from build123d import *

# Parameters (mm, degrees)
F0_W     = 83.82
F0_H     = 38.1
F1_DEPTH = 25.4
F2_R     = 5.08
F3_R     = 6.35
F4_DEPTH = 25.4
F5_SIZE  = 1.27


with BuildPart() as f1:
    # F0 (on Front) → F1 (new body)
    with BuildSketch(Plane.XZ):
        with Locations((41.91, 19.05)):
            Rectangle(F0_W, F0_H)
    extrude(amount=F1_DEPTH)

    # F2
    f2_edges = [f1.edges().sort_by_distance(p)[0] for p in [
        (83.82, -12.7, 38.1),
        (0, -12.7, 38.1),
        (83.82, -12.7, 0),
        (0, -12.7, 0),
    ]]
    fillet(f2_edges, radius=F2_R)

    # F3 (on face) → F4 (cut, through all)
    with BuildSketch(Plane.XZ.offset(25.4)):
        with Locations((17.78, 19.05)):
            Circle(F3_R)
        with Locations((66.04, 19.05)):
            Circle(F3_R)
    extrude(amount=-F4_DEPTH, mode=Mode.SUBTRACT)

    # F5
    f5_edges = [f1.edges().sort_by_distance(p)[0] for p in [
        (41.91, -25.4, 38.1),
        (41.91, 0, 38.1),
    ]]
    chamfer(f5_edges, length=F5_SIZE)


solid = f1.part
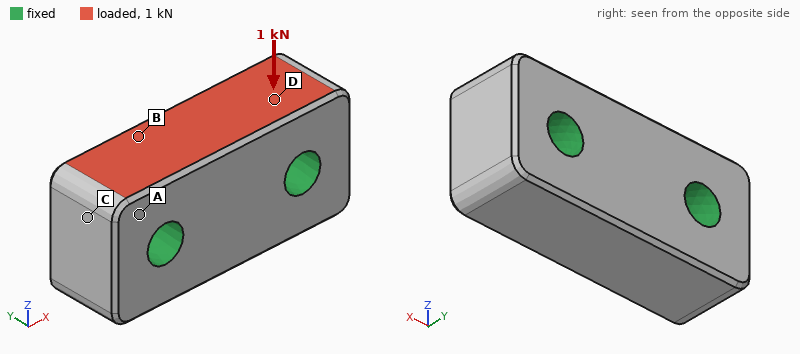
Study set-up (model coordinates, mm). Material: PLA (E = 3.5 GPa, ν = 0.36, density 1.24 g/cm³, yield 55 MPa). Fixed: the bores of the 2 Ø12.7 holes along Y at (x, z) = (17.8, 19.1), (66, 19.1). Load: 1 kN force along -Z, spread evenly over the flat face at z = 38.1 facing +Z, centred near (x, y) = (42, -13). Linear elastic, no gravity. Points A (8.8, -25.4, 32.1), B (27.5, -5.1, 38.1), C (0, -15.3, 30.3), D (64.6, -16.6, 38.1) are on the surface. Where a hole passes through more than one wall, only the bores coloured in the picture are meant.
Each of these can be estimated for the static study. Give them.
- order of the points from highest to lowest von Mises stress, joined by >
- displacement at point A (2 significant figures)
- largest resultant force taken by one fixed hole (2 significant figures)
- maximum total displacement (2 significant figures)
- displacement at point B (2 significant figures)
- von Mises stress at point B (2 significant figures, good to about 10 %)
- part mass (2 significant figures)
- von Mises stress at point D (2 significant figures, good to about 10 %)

D > B > A > C
1.7 µm
510 N
4.9 µm
3.6 µm
0.46 MPa
91 g
0.65 MPa
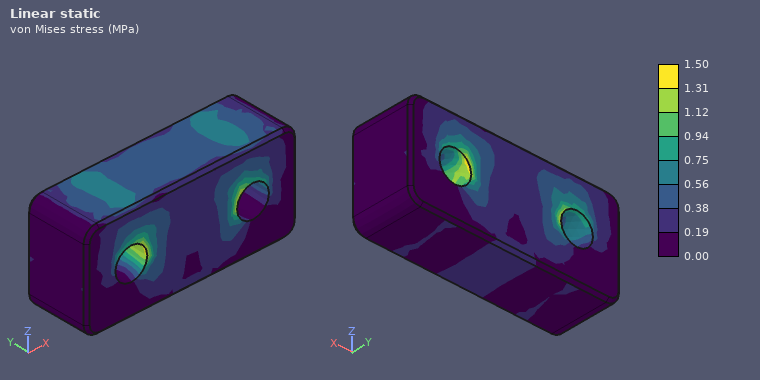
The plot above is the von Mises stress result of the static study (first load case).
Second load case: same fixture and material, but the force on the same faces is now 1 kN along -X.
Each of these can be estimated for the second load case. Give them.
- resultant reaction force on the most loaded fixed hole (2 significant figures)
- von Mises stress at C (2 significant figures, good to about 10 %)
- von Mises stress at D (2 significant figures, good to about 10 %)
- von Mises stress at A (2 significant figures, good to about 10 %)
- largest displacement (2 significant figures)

560 N
0.49 MPa
1.1 MPa
0.53 MPa
10 µm
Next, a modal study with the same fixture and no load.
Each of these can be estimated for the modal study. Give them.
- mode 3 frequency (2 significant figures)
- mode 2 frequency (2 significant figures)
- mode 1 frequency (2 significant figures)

9300 Hz
9200 Hz
9100 Hz
